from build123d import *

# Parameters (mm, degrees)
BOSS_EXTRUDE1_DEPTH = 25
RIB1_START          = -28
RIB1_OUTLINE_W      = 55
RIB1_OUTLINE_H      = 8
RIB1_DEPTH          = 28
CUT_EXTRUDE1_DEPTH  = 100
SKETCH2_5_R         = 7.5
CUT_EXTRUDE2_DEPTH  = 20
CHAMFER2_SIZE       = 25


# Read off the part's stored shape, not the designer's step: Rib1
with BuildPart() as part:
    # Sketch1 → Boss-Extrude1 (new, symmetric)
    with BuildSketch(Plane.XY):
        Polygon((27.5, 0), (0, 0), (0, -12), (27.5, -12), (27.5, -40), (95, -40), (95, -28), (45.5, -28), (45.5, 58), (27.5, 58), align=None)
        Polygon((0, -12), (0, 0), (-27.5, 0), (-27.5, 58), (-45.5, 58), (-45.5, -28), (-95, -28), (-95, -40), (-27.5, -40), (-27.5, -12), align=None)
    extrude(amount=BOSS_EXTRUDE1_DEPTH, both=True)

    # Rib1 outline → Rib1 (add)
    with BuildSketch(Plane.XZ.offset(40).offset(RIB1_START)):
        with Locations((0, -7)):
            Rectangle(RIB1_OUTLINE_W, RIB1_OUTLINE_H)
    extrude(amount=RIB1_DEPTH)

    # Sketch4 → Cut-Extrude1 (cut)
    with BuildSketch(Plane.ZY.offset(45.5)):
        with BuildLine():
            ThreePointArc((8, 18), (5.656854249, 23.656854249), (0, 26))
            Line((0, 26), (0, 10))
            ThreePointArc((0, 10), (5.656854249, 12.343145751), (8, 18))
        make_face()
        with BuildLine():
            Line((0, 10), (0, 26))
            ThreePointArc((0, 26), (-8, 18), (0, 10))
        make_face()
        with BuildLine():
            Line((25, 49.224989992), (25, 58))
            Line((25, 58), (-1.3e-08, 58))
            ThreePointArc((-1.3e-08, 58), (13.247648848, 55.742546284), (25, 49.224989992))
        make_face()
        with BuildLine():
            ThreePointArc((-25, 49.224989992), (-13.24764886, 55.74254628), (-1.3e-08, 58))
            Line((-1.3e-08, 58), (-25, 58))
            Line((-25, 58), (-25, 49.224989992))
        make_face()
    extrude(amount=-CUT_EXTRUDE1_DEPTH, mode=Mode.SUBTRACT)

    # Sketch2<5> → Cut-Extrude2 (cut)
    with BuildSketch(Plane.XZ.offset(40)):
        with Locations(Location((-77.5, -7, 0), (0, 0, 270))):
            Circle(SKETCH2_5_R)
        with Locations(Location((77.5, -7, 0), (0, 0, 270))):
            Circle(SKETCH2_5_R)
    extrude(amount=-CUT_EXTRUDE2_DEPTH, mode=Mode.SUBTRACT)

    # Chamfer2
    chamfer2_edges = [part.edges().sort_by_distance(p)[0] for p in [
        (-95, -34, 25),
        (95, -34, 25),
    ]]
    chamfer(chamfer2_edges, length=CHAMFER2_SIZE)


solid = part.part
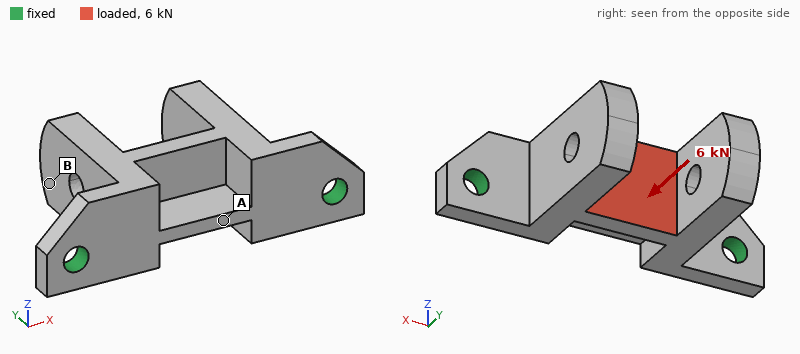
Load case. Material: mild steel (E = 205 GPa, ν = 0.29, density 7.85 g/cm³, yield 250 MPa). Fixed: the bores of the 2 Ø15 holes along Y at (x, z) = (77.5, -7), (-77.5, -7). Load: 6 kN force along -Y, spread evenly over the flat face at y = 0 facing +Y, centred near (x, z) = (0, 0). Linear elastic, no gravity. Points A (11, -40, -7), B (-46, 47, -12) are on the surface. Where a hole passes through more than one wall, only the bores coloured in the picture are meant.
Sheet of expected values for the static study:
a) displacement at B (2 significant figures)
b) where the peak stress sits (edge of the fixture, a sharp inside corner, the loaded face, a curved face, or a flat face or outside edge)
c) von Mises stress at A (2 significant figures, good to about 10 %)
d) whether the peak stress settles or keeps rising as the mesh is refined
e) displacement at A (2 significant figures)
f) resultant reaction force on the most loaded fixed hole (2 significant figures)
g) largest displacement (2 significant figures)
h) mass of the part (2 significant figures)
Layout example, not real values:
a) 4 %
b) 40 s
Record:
a) 20 µm
b) edge of the fixture
c) 13 MPa
d) keeps rising
e) 14 µm
f) 4.4 kN
g) 26 µm
h) 2.0 kg
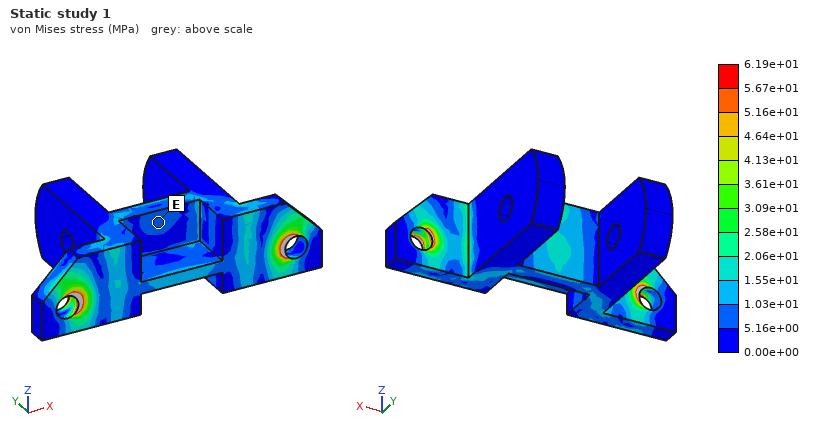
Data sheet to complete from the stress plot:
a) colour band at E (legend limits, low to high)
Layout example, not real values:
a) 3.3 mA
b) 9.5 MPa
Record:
a) 5.16e+00 to 1.03e+01 MPa
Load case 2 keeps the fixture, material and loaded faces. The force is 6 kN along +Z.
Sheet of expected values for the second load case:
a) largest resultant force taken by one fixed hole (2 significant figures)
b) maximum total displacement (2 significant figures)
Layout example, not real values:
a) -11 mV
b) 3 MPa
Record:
a) 3.0 kN
b) 0.14 mm
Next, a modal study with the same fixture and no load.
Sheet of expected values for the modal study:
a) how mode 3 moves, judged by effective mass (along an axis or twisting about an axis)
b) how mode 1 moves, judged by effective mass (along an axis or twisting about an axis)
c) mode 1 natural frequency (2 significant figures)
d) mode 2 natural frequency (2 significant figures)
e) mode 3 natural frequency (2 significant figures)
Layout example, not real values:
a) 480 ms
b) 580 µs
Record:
a) along X
b) along Z
c) 940 Hz
d) 1900 Hz
e) 2200 Hz
